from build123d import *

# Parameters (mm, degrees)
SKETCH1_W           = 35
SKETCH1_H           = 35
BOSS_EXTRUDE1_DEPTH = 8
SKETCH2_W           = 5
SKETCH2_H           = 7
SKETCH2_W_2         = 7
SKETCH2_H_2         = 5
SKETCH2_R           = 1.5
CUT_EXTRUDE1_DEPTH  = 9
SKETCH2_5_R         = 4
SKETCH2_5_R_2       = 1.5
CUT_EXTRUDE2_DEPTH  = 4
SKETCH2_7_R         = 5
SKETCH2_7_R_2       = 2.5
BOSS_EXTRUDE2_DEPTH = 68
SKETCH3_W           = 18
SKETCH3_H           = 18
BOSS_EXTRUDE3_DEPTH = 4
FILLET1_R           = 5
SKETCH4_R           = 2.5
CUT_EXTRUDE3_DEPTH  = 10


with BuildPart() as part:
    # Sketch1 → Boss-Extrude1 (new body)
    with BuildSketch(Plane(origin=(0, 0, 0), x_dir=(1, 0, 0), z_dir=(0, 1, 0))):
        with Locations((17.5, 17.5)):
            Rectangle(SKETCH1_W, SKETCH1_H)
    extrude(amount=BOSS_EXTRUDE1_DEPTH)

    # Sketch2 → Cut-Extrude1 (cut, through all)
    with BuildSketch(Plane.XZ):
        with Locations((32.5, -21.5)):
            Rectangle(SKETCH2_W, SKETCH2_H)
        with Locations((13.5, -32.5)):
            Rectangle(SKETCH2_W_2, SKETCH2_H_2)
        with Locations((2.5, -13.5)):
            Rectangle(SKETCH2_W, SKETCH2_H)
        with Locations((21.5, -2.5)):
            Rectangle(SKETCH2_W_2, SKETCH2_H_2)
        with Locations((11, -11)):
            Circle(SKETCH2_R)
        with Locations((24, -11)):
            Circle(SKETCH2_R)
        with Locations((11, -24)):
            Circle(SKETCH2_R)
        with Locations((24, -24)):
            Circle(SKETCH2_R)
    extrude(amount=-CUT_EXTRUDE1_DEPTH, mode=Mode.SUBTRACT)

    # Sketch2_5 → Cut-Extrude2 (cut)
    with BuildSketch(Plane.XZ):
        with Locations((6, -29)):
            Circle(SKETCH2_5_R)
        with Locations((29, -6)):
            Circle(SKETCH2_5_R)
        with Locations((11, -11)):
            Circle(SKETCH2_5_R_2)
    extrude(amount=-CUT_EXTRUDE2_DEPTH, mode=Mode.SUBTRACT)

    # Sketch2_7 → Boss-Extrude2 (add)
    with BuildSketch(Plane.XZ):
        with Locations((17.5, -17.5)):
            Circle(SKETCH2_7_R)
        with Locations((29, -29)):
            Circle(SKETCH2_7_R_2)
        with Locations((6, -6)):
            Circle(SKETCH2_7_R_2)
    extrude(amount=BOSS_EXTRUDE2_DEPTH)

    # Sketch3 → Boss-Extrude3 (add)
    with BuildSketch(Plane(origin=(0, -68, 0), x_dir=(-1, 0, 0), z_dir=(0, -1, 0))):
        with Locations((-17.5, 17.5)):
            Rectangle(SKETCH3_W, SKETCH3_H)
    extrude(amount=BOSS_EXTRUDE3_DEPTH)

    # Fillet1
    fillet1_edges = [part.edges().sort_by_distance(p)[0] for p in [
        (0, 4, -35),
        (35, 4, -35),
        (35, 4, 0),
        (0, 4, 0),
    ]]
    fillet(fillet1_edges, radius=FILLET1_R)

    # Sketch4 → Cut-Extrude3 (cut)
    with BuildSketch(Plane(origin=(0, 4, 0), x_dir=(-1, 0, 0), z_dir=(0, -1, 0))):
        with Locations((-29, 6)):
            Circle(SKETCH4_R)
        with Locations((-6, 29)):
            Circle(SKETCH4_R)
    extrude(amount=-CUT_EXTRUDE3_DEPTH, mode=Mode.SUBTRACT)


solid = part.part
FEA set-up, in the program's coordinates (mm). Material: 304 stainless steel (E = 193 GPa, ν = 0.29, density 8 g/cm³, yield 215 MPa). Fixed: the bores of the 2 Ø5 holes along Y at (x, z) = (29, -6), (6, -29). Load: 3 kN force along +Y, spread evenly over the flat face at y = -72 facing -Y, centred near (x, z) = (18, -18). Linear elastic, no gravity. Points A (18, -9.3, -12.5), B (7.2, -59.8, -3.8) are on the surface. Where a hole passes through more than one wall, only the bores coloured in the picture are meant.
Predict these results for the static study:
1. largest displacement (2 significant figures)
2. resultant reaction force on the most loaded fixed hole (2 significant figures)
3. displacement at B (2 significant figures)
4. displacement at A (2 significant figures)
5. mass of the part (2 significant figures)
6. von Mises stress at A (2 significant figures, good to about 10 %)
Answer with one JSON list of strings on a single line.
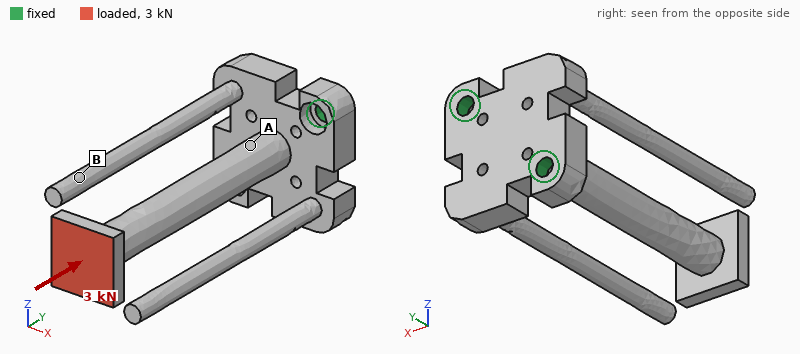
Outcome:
["26 µm", "1.8 kN", "12 µm", "9.1 µm", "140 g", "38 MPa"]
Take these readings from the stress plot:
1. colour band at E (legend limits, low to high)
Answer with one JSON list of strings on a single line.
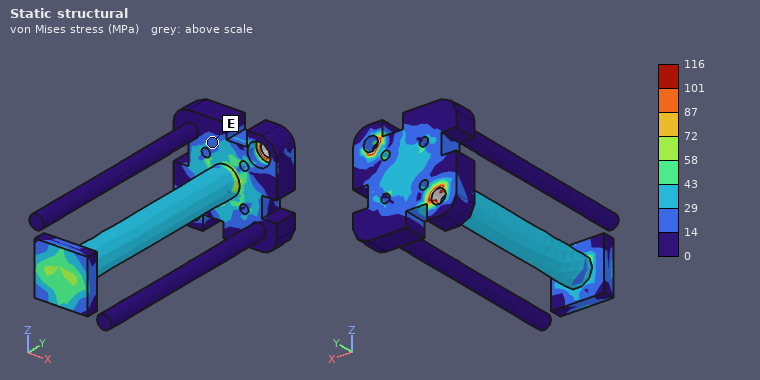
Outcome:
["14 to 29 MPa"]
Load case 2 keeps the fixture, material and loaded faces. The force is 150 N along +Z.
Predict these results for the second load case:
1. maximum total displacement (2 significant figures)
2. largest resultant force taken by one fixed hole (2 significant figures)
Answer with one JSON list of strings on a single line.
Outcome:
["0.27 mm", "310 N"]
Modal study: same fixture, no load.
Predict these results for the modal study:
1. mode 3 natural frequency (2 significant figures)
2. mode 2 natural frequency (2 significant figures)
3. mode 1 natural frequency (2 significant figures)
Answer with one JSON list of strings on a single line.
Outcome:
["710 Hz", "700 Hz", "670 Hz"]
